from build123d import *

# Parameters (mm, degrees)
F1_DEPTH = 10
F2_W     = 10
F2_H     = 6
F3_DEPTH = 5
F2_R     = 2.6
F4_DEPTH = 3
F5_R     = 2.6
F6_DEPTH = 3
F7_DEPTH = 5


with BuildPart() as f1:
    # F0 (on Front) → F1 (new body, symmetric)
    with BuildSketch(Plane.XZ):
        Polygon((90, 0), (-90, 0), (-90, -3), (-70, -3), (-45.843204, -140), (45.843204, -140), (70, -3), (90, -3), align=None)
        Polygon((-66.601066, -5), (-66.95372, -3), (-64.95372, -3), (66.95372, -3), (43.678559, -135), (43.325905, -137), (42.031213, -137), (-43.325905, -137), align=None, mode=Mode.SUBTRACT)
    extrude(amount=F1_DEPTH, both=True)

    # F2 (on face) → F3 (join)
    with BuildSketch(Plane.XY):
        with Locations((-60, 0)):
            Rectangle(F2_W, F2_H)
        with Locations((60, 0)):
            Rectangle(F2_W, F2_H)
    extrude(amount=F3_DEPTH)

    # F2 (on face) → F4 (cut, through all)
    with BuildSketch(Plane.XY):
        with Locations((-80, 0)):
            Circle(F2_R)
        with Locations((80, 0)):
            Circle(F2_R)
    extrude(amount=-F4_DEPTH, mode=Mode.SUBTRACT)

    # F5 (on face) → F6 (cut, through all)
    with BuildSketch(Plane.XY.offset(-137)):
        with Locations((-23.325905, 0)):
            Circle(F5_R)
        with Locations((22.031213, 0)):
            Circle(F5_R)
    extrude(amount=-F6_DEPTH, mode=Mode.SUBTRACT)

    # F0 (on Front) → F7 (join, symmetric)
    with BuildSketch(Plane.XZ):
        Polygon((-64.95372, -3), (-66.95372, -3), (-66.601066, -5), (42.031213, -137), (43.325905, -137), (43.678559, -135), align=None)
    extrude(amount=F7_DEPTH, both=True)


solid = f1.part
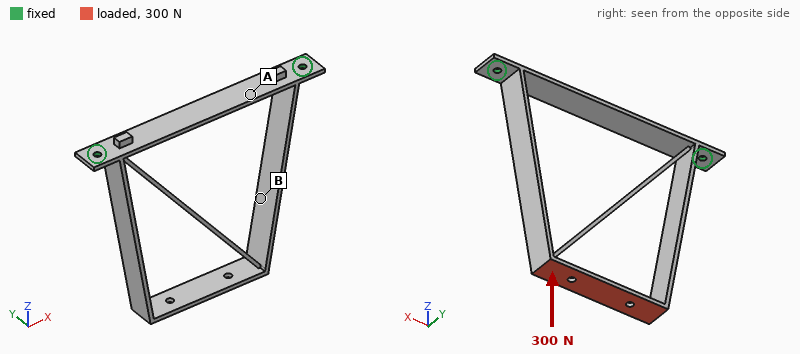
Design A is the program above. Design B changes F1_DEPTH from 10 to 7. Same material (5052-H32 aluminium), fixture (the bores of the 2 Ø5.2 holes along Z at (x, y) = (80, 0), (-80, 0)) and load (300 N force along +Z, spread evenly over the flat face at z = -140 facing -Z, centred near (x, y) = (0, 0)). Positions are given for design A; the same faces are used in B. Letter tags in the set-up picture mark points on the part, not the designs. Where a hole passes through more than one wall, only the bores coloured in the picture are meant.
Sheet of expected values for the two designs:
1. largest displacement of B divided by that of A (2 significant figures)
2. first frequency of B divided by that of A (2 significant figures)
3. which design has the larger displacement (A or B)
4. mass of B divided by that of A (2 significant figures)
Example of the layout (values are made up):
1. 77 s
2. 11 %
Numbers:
1. 1.4
2. 0.90
3. B
4. 0.74
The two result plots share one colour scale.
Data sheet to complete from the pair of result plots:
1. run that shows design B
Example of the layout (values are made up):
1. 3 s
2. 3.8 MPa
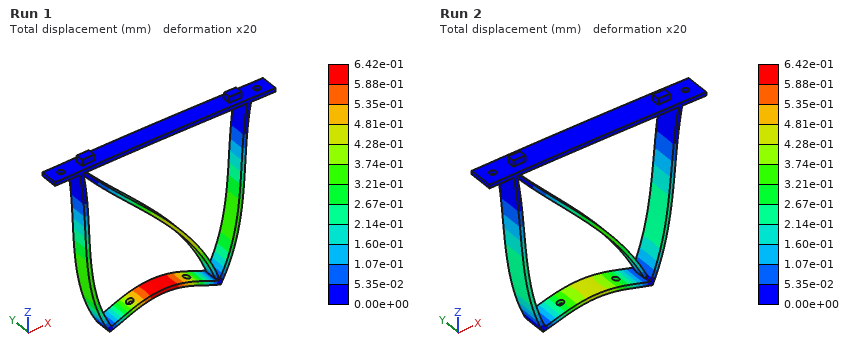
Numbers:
1. Run 1
